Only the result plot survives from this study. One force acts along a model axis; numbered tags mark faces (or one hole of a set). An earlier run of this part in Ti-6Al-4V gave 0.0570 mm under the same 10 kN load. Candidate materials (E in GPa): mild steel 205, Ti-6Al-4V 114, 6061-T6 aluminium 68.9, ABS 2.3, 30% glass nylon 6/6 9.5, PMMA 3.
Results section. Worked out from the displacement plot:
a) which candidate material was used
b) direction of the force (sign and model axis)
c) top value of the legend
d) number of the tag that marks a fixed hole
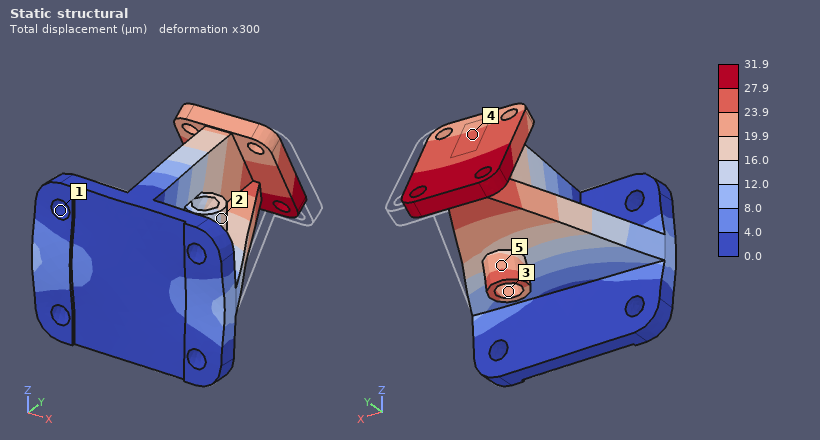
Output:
mild steel
-X
31.9 µm
1
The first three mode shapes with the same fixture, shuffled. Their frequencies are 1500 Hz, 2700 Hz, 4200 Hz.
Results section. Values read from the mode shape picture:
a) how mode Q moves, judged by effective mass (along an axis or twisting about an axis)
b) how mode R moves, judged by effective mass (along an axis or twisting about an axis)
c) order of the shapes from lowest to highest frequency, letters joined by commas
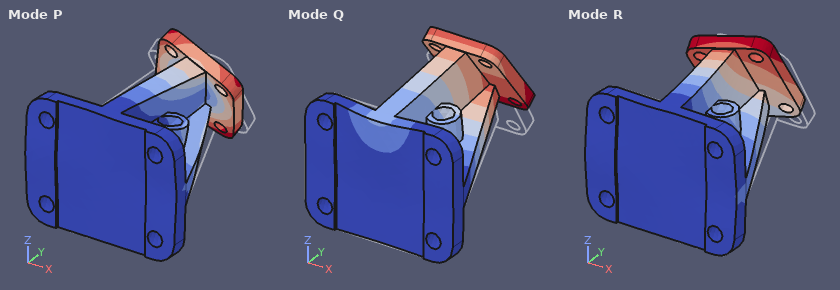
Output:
along Z
along X
Q, R, P
